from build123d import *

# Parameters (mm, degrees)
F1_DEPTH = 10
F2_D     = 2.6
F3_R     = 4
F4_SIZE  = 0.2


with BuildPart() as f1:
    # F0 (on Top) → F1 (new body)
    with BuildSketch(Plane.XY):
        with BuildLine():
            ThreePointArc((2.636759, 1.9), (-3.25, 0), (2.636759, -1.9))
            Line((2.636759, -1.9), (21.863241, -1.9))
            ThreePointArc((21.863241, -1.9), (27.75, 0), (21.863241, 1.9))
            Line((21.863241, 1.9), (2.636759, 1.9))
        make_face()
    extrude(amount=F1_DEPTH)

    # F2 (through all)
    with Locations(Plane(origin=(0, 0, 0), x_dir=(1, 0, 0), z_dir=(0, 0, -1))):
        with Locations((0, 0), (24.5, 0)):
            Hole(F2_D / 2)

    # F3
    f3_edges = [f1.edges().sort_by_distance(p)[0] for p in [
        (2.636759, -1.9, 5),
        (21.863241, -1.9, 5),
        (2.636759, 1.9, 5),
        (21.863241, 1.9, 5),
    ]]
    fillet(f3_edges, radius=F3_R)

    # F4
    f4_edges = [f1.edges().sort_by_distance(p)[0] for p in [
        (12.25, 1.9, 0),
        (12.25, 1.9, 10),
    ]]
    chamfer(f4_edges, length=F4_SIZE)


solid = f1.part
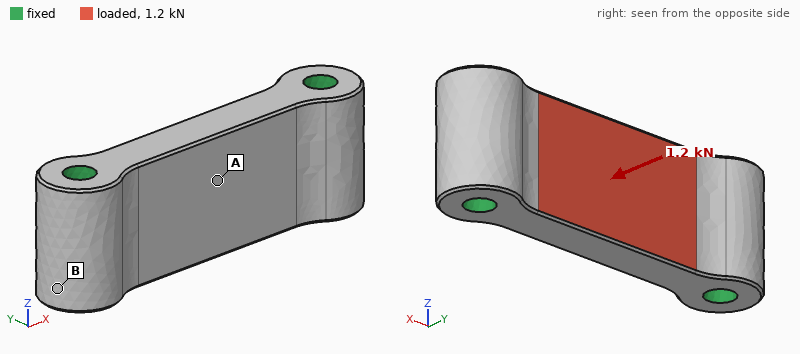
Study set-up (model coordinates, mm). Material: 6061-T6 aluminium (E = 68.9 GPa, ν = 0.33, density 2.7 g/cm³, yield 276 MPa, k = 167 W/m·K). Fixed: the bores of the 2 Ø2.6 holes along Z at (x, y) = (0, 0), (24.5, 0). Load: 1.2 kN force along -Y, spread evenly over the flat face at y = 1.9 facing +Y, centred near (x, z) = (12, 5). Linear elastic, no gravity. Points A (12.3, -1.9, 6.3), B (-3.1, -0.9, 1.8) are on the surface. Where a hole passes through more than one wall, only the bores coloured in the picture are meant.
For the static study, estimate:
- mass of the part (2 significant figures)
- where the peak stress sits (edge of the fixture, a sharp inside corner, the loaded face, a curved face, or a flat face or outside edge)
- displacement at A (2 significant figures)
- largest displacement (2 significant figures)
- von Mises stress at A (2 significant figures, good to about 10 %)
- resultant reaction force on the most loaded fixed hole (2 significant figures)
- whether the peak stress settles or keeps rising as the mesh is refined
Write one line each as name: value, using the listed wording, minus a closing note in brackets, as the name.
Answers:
mass of the part: 3.4 g
where the peak stress sits: edge of the fixture
displacement at A: 17 µm
largest displacement: 19 µm
von Mises stress at A: 56 MPa
resultant reaction force on the most loaded fixed hole: 600 N
whether the peak stress settles or keeps rising as the mesh is refined: keeps rising
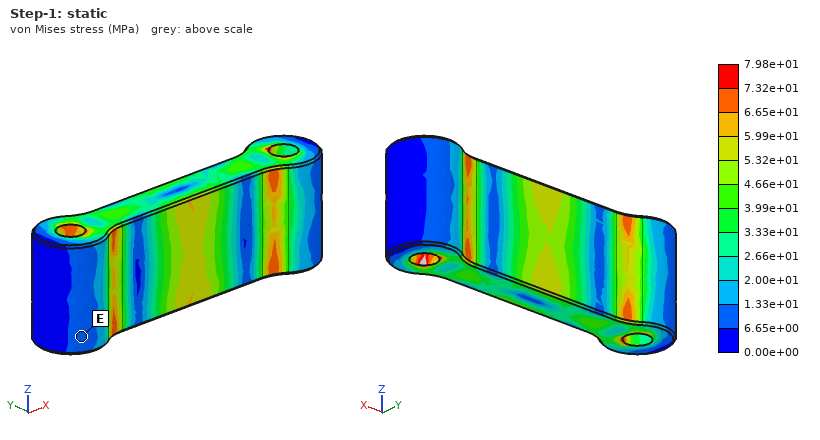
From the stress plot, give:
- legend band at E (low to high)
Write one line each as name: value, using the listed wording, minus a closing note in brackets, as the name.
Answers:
legend band at E: 6.65e+00 to 1.33e+01 MPa
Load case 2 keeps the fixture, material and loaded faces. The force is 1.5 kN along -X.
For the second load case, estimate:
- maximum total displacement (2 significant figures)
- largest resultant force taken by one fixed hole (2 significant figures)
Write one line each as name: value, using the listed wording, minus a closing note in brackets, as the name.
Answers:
maximum total displacement: 2.8 µm
largest resultant force taken by one fixed hole: 760 N
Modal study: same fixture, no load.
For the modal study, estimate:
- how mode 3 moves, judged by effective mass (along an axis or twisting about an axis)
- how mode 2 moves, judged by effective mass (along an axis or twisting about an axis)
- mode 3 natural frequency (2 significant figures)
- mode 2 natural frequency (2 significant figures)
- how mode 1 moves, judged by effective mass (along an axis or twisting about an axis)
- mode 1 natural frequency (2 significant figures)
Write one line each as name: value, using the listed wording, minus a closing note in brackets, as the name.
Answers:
how mode 3 moves, judged by effective mass: along Z
how mode 2 moves, judged by effective mass: twisting about X
mode 3 natural frequency: 56 kHz
mode 2 natural frequency: 53 kHz
how mode 1 moves, judged by effective mass: along Y
mode 1 natural frequency: 35 kHz
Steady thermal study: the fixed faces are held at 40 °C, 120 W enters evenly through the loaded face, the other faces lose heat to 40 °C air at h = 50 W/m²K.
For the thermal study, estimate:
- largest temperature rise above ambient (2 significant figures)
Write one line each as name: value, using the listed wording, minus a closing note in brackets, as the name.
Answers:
largest temperature rise above ambient: 71 K
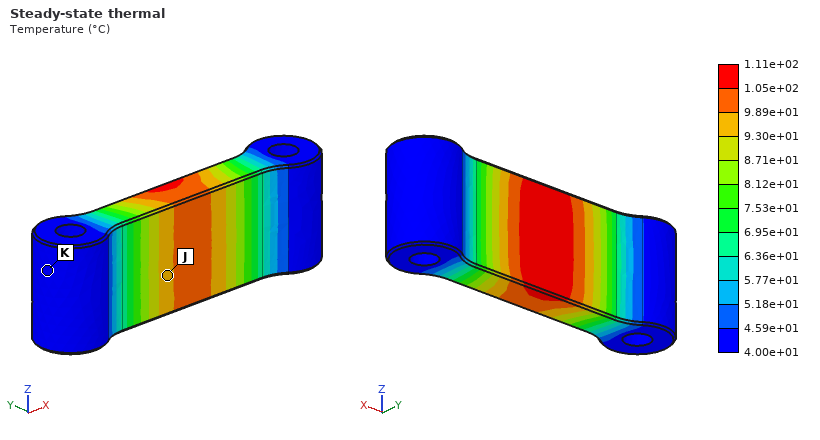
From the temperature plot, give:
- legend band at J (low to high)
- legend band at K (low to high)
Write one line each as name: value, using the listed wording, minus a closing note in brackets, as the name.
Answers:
legend band at J: 9.30e+01 to 9.89e+01 °C
legend band at K: 4.00e+01 to 4.59e+01 °C
